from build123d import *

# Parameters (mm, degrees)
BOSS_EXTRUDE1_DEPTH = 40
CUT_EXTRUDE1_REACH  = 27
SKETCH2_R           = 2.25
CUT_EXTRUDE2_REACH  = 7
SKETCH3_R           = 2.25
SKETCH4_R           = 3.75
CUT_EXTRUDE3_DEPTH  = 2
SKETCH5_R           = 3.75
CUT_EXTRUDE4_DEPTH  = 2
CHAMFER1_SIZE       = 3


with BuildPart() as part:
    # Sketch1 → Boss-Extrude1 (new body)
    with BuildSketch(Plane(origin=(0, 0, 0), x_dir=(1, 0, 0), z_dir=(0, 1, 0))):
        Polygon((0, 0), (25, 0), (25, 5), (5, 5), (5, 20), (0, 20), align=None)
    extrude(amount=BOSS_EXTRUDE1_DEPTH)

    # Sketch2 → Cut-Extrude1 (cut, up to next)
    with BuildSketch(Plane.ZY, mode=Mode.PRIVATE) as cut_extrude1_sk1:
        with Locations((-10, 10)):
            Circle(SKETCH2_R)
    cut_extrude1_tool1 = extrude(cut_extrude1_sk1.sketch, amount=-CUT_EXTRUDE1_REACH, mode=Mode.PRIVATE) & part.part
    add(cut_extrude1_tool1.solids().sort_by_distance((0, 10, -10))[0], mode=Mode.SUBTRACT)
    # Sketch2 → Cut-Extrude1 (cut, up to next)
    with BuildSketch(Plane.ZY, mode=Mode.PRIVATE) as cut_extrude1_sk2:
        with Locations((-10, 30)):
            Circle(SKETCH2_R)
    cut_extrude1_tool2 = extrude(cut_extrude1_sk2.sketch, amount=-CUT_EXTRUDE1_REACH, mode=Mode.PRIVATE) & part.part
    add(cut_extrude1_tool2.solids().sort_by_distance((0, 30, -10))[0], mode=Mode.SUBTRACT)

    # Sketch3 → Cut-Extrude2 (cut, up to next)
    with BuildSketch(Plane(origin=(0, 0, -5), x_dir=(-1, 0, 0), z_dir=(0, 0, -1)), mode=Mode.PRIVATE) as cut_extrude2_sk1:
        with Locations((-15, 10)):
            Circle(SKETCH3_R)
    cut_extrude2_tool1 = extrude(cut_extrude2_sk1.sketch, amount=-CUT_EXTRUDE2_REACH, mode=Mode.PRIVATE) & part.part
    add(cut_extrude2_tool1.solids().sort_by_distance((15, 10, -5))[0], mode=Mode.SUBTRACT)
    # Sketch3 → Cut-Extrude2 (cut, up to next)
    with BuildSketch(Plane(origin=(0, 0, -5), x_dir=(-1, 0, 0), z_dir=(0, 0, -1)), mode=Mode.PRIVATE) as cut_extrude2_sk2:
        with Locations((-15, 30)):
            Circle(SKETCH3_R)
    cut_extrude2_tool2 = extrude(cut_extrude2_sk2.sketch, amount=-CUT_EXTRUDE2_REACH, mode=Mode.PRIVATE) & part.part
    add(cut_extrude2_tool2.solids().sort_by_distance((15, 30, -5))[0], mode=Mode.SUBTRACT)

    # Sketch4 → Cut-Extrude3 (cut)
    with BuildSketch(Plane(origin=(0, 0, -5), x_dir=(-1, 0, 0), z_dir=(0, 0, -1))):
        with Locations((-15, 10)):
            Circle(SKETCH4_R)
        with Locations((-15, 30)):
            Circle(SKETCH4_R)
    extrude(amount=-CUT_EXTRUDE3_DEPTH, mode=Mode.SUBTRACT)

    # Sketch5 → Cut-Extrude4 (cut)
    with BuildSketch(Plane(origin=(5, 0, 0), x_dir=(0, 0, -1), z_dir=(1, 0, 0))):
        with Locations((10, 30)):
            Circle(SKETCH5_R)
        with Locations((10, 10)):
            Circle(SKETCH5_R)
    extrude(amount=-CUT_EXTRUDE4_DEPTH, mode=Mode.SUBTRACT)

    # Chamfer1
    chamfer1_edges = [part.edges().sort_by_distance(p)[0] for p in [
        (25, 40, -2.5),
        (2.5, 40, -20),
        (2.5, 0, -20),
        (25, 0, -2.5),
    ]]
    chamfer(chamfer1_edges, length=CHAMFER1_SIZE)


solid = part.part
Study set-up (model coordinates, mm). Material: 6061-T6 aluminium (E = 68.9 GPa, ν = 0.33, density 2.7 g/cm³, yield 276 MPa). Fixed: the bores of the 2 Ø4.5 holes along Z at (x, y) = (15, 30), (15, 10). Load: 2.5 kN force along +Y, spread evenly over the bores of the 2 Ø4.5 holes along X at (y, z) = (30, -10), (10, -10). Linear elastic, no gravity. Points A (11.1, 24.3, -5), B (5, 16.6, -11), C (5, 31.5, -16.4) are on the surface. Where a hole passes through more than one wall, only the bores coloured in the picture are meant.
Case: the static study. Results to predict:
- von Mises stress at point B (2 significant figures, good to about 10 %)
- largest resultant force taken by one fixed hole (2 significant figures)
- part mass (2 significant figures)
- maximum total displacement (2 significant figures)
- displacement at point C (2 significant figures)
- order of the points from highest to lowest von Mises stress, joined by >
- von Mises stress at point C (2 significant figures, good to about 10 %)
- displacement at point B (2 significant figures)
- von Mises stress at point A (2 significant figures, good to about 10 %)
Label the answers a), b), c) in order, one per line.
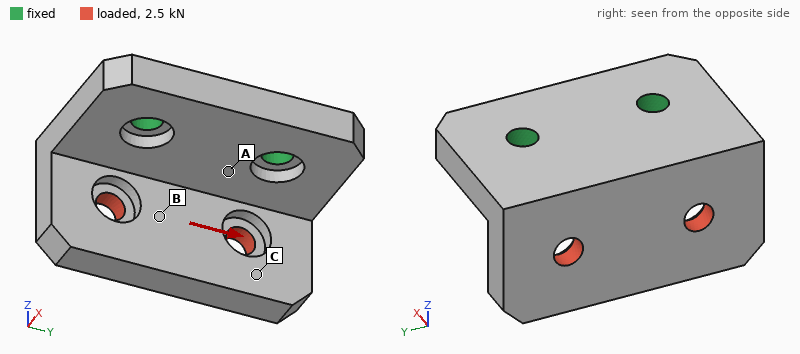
a) 36 MPa
b) 2.1 kN
c) 20 g
d) 69 µm
e) 55 µm
f) A > B > C
g) 17 MPa
h) 35 µm
i) 63 MPa
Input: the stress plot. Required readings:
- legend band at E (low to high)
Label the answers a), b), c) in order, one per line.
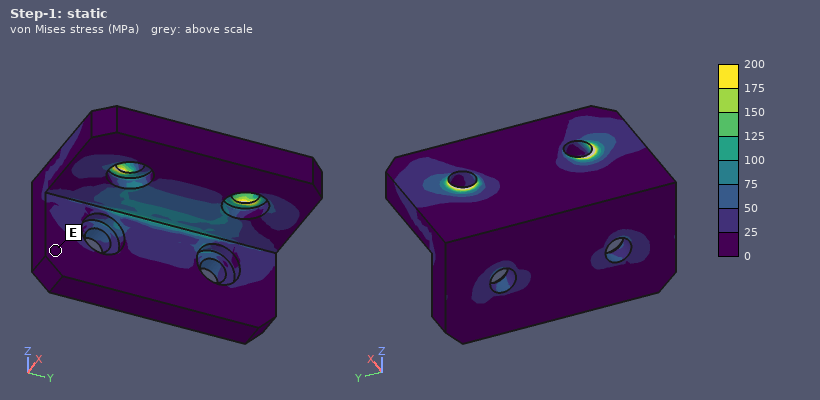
a) 0 to 25 MPa
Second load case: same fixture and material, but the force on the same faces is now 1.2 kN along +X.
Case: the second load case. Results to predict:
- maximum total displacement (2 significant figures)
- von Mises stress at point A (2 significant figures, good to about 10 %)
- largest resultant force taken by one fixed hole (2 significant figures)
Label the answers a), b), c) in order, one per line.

a) 0.13 mm
b) 63 MPa
c) 600 N
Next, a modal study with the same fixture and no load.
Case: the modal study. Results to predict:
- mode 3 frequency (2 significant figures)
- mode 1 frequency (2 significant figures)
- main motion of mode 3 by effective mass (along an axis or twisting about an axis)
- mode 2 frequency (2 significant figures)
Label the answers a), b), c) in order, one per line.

a) 14 kHz
b) 4800 Hz
c) along Z
d) 8100 Hz
